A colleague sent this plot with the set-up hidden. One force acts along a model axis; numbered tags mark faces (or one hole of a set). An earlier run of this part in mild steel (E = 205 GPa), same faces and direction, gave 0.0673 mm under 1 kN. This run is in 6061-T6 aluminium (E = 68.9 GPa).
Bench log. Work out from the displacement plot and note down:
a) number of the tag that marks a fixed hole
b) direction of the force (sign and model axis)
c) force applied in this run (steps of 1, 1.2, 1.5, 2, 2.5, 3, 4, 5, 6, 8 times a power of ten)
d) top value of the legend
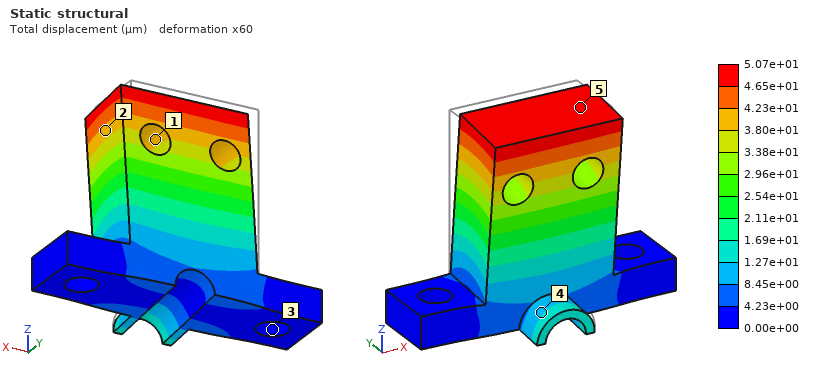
3
-Y
250 N
5.07e+01 µm
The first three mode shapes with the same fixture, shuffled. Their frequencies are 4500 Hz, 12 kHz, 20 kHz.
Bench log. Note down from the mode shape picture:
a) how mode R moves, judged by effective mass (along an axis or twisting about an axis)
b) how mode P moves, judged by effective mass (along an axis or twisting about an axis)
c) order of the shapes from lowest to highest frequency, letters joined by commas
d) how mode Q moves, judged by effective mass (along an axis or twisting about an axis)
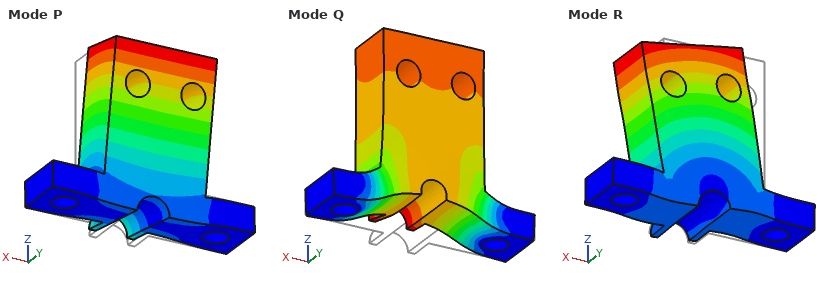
along X
along Y
P, R, Q
along Z
